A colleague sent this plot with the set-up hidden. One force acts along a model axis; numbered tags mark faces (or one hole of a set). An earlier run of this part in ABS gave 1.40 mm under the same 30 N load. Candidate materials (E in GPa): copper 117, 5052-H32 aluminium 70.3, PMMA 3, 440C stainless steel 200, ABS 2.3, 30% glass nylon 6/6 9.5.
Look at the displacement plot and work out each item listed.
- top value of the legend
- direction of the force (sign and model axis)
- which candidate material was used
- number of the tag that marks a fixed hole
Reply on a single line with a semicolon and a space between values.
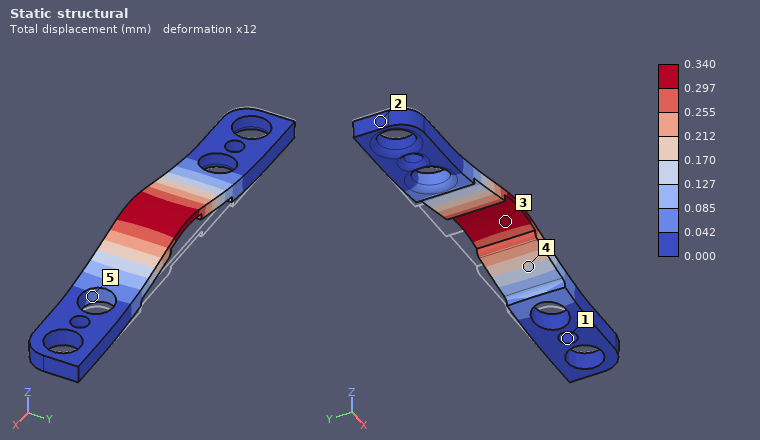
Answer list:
0.340 mm; +Z; 30% glass nylon 6/6; 1
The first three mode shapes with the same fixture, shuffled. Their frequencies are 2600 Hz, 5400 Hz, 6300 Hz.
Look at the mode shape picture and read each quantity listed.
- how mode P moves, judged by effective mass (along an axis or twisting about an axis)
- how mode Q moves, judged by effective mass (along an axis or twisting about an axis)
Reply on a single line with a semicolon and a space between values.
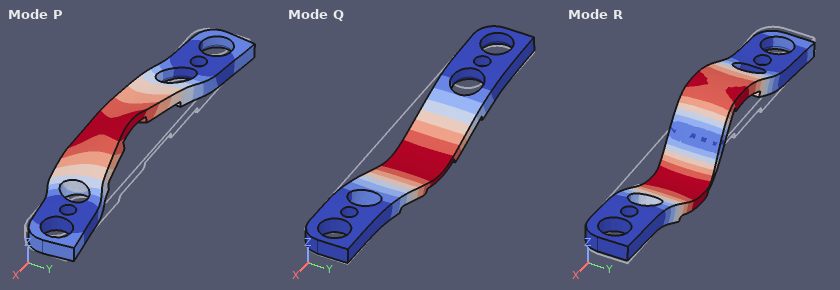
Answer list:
along Y; along Z
